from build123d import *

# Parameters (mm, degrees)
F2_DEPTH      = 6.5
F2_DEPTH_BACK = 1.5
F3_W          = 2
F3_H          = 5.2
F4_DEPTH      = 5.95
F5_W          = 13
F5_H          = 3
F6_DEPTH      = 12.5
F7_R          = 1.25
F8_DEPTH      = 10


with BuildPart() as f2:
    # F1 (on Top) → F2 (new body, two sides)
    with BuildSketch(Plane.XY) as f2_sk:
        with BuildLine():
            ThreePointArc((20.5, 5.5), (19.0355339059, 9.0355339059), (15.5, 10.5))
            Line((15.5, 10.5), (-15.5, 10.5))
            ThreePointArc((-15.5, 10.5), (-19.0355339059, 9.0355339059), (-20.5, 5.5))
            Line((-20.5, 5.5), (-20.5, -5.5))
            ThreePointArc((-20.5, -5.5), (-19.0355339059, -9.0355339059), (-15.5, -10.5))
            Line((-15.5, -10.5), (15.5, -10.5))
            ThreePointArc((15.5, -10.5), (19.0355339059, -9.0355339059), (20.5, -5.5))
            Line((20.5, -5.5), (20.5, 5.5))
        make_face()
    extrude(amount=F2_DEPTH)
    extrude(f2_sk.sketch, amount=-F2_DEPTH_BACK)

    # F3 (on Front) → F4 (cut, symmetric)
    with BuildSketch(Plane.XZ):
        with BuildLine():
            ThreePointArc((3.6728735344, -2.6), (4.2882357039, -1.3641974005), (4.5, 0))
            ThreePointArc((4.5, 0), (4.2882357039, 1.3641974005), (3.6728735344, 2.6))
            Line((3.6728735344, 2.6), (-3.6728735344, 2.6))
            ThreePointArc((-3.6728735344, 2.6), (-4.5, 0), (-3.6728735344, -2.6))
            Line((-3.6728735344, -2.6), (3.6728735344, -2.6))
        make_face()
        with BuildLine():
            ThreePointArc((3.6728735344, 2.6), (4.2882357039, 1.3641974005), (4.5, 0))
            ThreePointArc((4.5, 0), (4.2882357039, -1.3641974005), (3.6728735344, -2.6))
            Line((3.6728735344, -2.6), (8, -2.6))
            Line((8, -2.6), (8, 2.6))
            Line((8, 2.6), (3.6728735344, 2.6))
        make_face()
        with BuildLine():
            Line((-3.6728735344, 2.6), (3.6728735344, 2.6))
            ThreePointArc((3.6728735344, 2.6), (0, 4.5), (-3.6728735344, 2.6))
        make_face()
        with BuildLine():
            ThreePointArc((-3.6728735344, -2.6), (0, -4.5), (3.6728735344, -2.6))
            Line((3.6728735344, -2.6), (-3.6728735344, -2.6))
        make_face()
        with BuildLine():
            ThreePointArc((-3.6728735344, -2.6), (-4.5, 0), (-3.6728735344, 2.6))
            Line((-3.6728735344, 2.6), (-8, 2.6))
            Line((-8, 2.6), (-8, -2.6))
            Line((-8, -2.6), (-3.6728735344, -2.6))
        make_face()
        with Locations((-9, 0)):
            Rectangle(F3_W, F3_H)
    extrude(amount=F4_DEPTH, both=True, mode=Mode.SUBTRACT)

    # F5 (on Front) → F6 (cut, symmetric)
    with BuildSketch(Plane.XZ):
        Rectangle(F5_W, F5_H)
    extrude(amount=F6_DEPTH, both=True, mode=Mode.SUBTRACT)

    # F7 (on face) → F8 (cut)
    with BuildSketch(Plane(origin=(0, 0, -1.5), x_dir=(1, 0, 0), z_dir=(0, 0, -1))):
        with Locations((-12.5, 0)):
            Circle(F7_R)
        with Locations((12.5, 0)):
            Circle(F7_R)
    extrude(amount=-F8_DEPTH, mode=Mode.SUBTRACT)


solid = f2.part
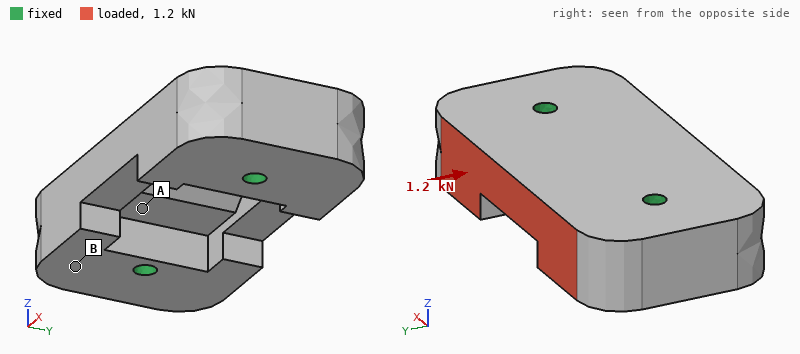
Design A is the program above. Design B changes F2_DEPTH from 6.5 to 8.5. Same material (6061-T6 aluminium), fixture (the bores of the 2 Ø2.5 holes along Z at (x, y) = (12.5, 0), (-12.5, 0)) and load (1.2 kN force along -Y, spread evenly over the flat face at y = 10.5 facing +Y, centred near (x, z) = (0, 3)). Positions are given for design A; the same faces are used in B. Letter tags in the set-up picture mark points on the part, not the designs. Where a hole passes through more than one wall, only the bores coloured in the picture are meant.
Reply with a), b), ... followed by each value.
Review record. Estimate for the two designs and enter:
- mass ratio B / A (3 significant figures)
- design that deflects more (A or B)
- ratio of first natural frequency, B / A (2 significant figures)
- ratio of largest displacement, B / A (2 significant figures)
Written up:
a) 1.31
b) A
c) 1.1
d) 0.72
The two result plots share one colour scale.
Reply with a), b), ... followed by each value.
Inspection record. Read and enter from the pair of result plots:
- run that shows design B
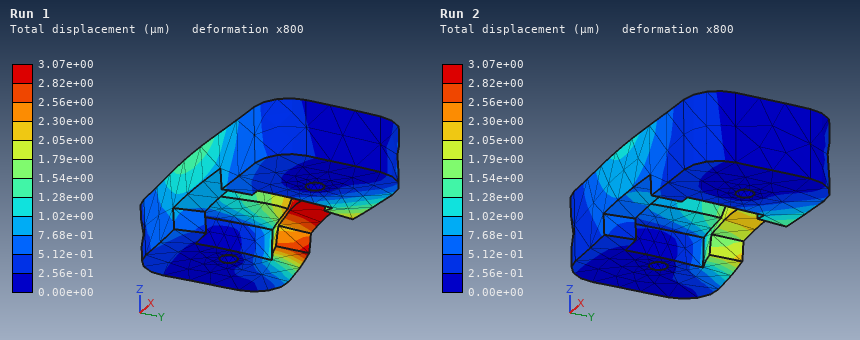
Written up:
a) Run 2
